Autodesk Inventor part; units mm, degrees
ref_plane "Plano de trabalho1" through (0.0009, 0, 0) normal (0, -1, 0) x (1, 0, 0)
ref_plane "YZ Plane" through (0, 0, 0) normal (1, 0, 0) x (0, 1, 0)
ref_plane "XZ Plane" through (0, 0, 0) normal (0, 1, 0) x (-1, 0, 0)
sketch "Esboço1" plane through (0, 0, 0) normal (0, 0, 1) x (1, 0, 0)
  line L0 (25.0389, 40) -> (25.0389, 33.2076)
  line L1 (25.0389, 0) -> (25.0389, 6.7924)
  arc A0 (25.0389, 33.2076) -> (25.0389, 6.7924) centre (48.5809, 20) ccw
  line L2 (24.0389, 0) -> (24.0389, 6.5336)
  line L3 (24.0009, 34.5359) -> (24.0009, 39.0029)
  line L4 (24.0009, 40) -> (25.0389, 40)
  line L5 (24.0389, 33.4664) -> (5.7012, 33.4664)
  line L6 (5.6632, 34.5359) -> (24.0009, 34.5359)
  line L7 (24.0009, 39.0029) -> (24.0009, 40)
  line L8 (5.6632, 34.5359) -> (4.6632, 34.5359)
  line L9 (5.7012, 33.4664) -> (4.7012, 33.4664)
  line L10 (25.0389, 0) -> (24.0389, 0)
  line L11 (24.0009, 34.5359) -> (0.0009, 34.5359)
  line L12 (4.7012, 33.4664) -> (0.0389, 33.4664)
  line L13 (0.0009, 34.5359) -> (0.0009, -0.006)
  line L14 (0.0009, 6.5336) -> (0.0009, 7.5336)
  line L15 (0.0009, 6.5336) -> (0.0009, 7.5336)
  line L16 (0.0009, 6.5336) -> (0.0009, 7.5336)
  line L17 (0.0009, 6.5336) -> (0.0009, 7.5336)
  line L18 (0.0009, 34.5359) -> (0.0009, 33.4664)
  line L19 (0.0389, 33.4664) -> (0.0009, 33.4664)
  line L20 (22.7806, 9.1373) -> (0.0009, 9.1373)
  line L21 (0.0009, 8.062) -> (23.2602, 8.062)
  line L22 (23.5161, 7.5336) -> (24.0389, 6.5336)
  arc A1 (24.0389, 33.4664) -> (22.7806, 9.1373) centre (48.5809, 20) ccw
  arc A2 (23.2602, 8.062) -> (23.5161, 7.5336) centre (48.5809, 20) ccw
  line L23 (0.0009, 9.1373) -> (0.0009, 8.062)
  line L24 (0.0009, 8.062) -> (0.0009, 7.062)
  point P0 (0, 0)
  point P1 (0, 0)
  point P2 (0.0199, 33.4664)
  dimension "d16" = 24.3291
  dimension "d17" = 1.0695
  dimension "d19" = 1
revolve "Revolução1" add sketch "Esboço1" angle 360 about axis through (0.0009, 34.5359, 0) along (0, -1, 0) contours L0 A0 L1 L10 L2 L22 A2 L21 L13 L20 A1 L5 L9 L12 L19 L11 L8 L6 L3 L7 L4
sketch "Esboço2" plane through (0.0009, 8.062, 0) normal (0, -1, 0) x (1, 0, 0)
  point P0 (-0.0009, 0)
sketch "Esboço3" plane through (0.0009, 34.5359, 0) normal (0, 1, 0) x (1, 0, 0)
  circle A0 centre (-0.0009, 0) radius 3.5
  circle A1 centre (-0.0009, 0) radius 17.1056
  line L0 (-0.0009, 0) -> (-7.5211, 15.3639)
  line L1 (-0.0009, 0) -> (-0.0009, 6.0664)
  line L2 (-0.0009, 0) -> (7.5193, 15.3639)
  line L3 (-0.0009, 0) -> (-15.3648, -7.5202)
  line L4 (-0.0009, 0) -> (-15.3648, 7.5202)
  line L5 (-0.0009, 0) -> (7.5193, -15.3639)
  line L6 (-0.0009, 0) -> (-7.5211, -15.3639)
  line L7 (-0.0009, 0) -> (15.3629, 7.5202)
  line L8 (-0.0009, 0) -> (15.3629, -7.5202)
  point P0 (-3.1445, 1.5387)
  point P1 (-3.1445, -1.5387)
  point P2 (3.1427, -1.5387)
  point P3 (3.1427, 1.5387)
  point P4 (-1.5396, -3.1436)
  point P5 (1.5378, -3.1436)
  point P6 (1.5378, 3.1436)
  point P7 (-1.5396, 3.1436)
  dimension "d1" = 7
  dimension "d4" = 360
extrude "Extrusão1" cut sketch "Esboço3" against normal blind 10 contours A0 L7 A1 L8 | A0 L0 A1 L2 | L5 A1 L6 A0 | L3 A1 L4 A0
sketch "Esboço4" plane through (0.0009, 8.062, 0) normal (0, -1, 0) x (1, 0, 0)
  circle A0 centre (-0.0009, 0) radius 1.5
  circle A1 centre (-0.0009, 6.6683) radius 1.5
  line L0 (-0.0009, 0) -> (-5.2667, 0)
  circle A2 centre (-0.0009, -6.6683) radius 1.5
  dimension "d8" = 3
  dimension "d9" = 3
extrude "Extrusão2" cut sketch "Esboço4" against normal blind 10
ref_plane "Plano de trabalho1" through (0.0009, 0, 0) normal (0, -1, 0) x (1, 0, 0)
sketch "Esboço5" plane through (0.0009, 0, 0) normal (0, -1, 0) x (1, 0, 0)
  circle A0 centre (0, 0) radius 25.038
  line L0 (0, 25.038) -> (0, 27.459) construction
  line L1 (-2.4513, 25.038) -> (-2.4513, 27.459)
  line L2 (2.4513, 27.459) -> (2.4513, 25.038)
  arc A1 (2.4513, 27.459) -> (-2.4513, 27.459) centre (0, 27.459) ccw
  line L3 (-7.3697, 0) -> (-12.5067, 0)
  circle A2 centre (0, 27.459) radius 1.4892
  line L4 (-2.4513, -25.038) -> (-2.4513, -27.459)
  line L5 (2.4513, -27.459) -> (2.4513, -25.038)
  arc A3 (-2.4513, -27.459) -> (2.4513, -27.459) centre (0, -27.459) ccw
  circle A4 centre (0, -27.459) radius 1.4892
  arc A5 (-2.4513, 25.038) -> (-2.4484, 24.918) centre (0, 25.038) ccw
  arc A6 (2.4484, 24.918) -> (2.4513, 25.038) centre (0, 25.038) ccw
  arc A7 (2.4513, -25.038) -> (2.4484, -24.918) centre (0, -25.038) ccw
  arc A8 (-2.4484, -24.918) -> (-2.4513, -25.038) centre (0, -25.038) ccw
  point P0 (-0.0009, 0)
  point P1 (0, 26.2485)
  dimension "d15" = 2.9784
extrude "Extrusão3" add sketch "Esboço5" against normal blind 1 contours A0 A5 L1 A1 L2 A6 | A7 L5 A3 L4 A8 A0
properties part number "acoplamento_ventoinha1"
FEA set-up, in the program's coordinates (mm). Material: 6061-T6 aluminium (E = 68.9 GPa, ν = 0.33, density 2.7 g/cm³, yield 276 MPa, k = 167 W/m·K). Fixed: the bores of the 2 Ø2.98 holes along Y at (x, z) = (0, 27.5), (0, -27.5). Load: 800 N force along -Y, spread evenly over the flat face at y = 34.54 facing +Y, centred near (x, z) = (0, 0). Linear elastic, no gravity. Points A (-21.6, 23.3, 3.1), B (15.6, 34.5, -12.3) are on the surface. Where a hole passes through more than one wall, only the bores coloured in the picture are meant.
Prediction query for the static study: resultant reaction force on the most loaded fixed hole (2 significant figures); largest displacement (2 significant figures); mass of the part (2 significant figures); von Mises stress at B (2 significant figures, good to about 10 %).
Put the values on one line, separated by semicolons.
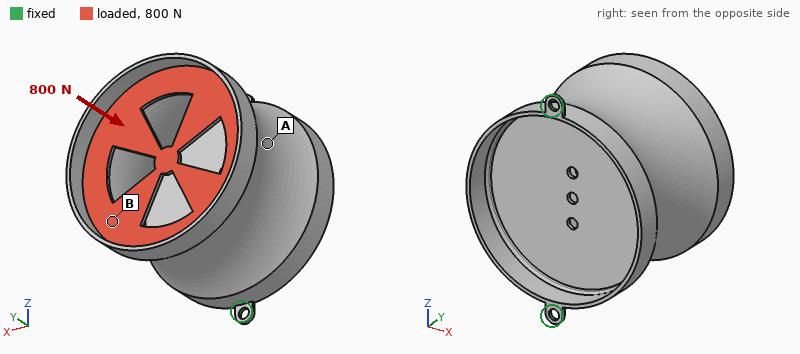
420 N; 0.57 mm; 25 g; 100 MPa
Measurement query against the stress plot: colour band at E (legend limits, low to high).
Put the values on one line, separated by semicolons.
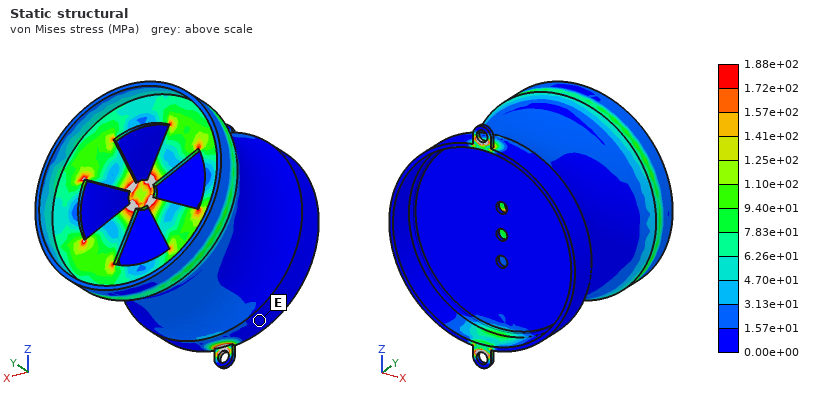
0.00e+00 to 1.57e+01 MPa
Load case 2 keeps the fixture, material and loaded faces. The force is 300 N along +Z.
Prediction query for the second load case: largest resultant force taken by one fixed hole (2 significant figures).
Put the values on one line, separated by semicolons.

250 N
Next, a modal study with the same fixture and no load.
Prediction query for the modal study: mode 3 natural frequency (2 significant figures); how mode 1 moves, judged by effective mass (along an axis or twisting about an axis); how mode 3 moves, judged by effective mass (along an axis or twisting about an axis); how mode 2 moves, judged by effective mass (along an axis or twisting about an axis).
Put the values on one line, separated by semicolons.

3800 Hz; along X; along Y; along Z
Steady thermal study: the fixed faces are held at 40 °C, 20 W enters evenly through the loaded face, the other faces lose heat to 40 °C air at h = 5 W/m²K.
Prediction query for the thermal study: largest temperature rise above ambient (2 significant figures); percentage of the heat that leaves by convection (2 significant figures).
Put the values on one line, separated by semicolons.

80 K; 24 %
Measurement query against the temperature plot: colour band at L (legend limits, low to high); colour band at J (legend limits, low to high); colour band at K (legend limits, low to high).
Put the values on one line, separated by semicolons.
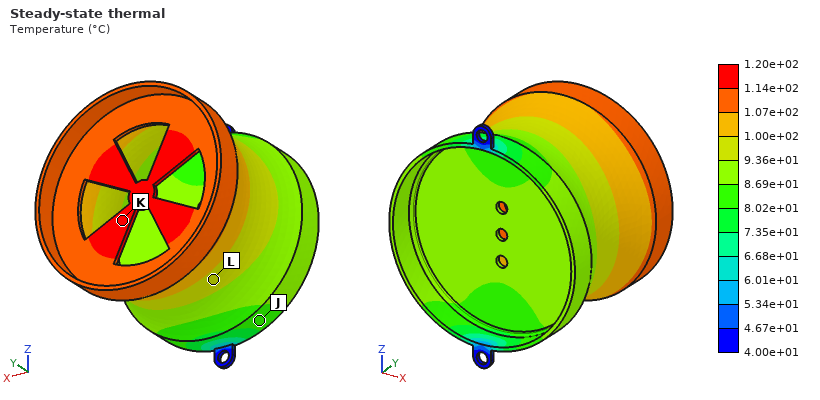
9.36e+01 to 1.00e+02 °C; 8.02e+01 to 8.69e+01 °C; 1.14e+02 to 1.20e+02 °C
